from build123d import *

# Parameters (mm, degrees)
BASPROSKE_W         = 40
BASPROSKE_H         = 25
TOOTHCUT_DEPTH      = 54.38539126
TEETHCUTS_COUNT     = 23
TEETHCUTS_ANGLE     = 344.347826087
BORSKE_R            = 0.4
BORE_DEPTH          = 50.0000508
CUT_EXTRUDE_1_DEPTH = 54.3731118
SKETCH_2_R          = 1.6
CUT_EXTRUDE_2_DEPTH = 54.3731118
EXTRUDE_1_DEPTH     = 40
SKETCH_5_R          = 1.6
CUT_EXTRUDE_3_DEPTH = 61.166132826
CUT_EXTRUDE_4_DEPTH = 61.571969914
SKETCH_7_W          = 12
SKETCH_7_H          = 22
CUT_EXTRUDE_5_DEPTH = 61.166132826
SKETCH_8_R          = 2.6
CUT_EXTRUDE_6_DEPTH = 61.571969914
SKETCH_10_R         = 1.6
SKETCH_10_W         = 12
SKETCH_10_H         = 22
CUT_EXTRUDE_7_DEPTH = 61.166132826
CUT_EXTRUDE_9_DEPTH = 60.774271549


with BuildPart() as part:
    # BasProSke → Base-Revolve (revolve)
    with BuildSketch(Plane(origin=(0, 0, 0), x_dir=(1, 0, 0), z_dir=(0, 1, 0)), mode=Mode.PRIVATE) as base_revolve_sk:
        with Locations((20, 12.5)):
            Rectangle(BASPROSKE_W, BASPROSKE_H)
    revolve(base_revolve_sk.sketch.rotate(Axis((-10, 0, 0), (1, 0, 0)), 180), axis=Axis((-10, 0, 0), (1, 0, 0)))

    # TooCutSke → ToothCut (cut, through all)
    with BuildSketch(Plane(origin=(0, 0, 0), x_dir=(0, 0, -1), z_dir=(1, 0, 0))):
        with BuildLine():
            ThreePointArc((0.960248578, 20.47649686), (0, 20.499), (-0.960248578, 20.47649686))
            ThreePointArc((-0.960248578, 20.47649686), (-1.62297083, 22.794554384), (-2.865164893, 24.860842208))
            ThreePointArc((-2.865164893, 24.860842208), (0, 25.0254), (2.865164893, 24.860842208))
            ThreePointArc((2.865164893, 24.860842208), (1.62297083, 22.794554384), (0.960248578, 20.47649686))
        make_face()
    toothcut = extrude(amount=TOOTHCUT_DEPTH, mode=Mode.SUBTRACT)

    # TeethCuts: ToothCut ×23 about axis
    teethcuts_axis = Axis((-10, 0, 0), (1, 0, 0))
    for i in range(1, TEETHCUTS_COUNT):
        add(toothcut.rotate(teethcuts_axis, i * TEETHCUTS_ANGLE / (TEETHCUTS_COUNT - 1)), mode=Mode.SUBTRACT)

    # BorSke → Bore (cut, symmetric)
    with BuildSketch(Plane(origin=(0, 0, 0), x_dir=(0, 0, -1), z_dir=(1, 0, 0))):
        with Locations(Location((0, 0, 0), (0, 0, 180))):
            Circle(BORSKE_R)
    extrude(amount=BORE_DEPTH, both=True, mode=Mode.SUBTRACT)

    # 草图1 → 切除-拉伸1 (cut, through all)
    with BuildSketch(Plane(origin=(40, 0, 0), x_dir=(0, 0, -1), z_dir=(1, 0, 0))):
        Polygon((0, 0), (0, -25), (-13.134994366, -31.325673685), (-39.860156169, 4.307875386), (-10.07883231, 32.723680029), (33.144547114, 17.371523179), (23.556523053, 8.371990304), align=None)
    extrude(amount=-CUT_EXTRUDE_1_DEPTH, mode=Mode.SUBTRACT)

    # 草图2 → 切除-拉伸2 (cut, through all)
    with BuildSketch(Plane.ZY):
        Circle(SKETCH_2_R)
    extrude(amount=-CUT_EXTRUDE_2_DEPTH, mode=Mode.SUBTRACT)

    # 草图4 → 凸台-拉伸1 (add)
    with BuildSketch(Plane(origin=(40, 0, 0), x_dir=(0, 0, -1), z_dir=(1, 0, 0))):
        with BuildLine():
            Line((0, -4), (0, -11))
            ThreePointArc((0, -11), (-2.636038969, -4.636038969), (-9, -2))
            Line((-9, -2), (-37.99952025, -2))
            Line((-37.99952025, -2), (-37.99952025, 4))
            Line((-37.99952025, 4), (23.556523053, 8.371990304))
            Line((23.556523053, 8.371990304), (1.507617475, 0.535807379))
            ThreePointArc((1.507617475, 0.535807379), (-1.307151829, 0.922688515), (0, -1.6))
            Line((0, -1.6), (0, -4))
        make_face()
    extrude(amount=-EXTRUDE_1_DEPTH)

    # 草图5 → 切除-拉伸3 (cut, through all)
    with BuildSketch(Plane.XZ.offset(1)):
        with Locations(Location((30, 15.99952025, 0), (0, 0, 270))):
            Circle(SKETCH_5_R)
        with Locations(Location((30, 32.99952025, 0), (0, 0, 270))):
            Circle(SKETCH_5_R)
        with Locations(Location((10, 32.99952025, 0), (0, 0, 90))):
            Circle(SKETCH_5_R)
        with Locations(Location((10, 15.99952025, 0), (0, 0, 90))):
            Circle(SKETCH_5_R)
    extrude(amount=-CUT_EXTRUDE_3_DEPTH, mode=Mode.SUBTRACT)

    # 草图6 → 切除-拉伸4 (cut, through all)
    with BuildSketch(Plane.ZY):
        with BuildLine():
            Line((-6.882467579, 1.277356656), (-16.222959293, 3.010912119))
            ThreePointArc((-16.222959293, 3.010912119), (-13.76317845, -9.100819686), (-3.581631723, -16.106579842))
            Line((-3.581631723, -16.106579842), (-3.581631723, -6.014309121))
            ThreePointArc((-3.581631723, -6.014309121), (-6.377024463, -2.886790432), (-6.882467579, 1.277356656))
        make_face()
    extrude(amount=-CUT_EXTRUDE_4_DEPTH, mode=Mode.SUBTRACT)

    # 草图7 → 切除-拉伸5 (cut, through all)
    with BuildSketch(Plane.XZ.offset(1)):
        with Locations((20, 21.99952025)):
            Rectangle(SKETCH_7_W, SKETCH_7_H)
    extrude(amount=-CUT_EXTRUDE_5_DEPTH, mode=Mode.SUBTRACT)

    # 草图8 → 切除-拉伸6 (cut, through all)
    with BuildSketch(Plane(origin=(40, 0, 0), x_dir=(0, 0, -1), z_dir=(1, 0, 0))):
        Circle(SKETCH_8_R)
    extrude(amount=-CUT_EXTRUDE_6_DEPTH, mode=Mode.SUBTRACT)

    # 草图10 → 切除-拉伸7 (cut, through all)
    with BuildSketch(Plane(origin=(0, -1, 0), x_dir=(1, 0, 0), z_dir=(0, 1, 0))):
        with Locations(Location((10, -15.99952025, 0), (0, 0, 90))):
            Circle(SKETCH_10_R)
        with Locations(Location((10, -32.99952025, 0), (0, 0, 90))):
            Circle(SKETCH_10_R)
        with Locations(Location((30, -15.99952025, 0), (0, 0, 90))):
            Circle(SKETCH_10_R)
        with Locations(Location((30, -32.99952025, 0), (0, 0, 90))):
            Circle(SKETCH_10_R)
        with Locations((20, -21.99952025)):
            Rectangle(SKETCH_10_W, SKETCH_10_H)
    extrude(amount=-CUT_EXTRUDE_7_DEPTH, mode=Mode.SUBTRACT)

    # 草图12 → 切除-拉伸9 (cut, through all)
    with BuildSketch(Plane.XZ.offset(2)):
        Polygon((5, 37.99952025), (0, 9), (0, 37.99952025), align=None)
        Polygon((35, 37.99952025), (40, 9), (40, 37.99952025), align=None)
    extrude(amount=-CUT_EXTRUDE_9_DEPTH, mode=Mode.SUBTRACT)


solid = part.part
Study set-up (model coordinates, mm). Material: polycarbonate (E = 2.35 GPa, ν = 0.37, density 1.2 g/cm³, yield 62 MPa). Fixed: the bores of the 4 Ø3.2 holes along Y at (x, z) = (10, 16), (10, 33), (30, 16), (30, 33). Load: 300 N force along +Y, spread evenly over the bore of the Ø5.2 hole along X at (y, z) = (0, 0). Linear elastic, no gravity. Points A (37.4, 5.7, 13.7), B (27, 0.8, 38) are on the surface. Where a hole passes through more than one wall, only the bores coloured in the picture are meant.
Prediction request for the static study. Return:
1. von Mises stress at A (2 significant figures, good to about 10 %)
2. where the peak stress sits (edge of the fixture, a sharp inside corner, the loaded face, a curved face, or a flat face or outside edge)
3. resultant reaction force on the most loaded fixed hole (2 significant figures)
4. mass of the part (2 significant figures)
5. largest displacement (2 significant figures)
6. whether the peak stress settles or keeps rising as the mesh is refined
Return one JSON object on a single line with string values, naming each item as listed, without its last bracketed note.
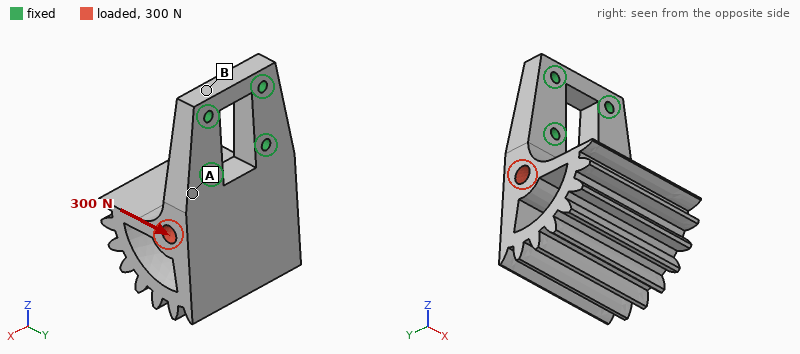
{"von Mises stress at A": "8.4 MPa", "where the peak stress sits": "edge of the fixture", "resultant reaction force on the most loaded fixed hole": "180 N", "mass of the part": "29 g", "largest displacement": "0.59 mm", "whether the peak stress settles or keeps rising as the mesh is refined": "keeps rising"}
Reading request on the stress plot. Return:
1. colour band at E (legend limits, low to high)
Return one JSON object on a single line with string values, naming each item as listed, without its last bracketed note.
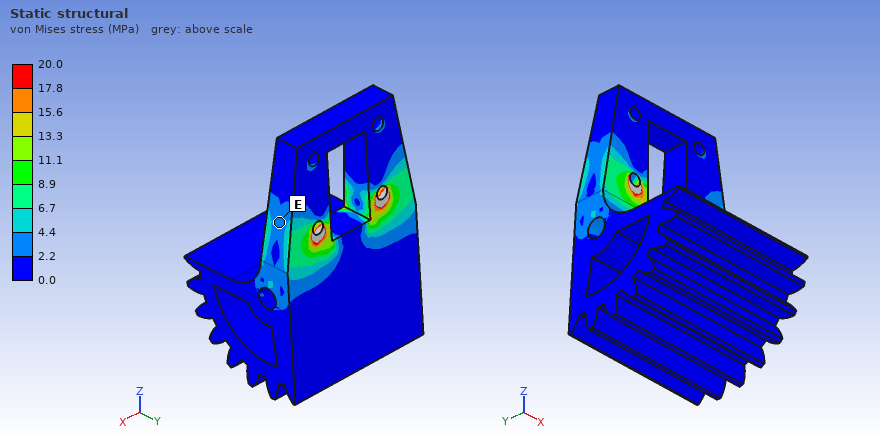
{"colour band at E": "2.2 to 4.4 MPa"}
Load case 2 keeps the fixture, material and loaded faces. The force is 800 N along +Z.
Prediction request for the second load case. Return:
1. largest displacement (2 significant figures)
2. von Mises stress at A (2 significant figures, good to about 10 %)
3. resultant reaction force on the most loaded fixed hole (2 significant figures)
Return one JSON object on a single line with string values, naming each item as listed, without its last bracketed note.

{"largest displacement": "0.28 mm", "von Mises stress at A": "2.1 MPa", "resultant reaction force on the most loaded fixed hole": "360 N"}
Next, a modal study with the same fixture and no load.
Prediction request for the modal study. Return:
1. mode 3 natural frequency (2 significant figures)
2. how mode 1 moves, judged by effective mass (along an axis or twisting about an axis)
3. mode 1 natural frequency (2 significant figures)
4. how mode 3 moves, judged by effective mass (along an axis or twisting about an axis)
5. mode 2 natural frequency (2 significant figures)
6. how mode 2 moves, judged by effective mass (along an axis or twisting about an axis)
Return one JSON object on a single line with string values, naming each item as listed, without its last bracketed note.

{"mode 3 natural frequency": "2300 Hz", "how mode 1 moves, judged by effective mass": "along Y", "mode 1 natural frequency": "600 Hz", "how mode 3 moves, judged by effective mass": "along X", "mode 2 natural frequency": "1500 Hz", "how mode 2 moves, judged by effective mass": "along X"}
